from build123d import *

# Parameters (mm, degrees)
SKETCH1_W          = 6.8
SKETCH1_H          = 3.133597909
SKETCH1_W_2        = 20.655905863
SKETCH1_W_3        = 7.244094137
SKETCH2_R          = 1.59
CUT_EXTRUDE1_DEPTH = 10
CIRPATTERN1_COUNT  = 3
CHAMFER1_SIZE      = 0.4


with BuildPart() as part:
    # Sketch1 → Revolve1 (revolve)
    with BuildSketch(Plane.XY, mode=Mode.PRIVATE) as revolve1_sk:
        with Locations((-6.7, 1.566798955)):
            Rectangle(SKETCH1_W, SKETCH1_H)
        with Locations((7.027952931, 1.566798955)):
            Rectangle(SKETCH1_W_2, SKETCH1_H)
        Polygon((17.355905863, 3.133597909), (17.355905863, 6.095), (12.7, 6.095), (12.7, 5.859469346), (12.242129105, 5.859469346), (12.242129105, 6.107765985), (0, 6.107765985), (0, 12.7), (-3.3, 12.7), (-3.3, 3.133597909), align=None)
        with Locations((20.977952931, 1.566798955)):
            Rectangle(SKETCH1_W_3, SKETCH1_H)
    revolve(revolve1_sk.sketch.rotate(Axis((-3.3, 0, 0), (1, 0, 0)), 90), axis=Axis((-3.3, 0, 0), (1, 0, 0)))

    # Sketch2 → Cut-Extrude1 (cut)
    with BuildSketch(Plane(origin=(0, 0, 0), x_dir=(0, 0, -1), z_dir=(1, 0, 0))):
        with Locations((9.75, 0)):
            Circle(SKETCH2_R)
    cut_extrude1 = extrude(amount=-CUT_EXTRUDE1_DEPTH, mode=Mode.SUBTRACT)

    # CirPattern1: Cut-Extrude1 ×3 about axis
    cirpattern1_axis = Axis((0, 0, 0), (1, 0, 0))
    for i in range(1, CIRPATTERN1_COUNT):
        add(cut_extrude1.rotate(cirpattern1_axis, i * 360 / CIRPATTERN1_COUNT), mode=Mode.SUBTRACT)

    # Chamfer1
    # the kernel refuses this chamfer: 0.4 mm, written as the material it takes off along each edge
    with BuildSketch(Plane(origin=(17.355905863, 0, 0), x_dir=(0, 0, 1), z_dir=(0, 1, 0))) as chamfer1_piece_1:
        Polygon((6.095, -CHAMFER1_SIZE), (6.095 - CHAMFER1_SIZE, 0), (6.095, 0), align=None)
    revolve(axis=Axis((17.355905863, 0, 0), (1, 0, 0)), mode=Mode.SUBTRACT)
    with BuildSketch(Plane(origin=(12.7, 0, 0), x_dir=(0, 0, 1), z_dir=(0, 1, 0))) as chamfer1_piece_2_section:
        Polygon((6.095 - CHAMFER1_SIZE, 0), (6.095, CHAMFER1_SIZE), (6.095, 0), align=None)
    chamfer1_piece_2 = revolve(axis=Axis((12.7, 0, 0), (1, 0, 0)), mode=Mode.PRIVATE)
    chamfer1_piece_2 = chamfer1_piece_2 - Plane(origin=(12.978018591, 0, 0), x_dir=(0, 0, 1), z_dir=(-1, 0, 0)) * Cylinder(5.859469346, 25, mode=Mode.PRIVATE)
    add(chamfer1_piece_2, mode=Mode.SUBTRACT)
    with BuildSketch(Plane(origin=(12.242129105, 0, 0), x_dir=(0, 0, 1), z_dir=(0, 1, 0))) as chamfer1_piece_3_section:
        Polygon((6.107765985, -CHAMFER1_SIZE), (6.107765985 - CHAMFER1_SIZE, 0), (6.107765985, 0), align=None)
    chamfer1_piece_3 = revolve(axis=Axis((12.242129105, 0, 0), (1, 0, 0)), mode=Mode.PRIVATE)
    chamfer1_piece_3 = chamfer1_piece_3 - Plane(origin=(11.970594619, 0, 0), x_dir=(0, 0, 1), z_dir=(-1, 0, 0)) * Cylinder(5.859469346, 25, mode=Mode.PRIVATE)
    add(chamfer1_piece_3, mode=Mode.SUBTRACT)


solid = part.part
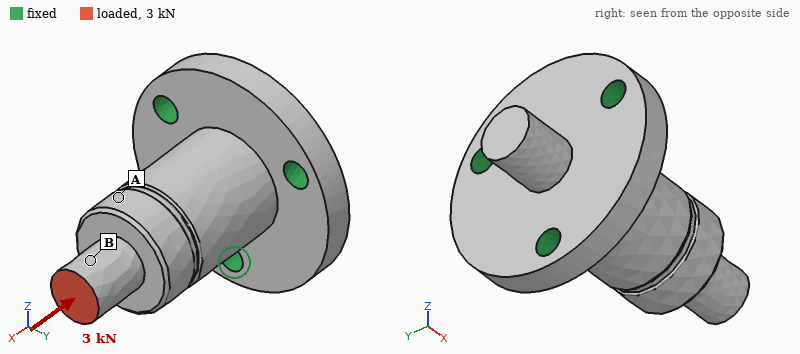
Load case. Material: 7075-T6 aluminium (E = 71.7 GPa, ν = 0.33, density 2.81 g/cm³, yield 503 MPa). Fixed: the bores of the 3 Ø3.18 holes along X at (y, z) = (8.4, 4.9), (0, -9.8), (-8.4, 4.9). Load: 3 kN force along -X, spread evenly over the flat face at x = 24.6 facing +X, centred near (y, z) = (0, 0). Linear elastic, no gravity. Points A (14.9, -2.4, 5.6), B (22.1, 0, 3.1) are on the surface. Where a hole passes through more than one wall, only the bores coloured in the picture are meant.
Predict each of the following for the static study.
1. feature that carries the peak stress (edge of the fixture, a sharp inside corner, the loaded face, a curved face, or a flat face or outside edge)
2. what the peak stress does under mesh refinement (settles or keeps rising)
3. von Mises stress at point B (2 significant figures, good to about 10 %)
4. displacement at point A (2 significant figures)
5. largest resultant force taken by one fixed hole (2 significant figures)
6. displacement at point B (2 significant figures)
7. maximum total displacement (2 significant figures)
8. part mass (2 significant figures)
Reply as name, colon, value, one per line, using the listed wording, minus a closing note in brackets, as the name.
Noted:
feature that carries the peak stress: edge of the fixture
what the peak stress does under mesh refinement: keeps rising
von Mises stress at point B: 96 MPa
displacement at point A: 14 µm
largest resultant force taken by one fixed hole: 1.0 kN
displacement at point B: 24 µm
maximum total displacement: 27 µm
part mass: 11 g
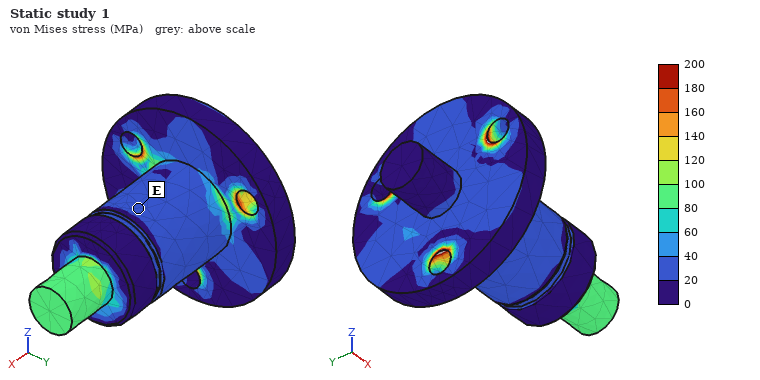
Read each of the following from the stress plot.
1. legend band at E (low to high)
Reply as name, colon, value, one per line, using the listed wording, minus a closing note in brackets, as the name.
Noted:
legend band at E: 20 to 40 MPa
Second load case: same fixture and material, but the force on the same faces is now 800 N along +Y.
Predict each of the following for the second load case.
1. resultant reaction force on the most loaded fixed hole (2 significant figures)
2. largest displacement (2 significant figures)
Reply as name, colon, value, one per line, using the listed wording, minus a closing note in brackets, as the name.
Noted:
resultant reaction force on the most loaded fixed hole: 1.4 kN
largest displacement: 0.15 mm
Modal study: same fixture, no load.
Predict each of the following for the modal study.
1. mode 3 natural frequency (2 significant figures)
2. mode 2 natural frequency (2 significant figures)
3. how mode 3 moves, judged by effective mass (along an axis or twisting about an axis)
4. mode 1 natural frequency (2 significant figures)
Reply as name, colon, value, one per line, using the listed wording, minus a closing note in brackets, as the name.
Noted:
mode 3 natural frequency: 28 kHz
mode 2 natural frequency: 12 kHz
how mode 3 moves, judged by effective mass: along X
mode 1 natural frequency: 12 kHz
